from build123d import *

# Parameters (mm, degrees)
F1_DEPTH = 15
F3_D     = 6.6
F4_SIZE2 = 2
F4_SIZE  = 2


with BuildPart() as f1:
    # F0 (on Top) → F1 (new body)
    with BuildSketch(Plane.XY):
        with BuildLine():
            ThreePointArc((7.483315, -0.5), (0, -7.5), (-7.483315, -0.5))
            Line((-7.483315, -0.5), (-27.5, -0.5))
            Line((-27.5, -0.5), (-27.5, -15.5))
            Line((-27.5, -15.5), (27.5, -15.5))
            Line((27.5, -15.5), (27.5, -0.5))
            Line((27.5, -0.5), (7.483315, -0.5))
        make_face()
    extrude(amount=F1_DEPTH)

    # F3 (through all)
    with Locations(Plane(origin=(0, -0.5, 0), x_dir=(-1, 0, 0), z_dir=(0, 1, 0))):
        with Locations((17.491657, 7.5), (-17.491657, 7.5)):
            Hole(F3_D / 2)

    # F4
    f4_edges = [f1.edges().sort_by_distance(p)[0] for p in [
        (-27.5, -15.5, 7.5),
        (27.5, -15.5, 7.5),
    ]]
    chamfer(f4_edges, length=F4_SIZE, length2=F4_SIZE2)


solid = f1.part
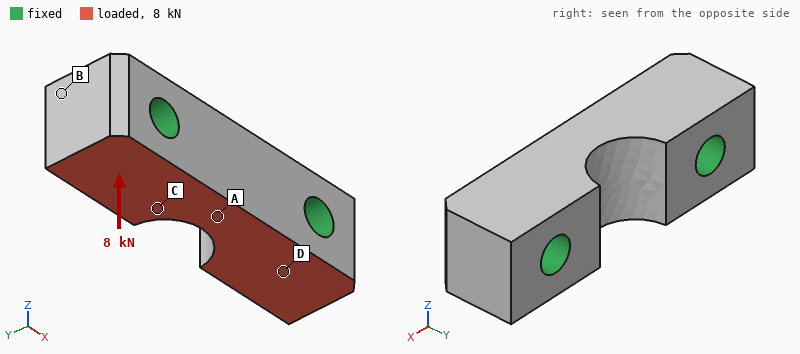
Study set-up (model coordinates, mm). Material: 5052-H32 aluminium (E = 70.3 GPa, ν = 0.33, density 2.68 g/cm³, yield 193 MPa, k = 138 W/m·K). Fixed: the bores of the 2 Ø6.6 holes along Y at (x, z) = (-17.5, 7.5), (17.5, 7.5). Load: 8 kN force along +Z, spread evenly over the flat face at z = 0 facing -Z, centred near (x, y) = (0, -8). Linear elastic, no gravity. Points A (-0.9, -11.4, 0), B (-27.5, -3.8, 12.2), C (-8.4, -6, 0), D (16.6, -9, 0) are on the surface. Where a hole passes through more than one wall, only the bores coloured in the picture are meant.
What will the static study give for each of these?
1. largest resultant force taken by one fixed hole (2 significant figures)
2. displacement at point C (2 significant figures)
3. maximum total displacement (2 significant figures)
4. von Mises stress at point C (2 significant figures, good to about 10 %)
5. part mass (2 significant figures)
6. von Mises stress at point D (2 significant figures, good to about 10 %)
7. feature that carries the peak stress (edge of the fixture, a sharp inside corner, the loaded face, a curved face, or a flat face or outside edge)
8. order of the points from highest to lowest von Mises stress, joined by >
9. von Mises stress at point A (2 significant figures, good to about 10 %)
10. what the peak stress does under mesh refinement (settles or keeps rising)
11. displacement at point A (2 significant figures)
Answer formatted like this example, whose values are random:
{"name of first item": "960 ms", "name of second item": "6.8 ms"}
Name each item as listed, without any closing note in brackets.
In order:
{"largest resultant force taken by one fixed hole": "4.0 kN", "displacement at point C": "4.2 µm", "maximum total displacement": "6.9 µm", "von Mises stress at point C": "9.1 MPa", "part mass": "27 g", "von Mises stress at point D": "25 MPa", "feature that carries the peak stress": "edge of the fixture", "order of the points from highest to lowest von Mises stress, joined by >": "D > A > C > B", "von Mises stress at point A": "16 MPa", "what the peak stress does under mesh refinement": "keeps rising", "displacement at point A": "6.0 µm"}
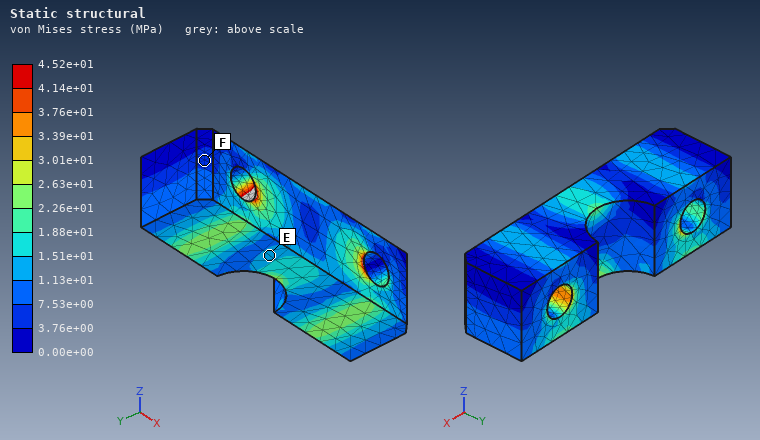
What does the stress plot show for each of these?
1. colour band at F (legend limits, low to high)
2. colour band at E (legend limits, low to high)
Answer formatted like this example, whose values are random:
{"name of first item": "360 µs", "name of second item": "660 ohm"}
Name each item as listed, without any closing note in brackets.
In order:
{"colour band at F": "3.76e+00 to 7.53e+00 MPa", "colour band at E": "1.13e+01 to 1.51e+01 MPa"}
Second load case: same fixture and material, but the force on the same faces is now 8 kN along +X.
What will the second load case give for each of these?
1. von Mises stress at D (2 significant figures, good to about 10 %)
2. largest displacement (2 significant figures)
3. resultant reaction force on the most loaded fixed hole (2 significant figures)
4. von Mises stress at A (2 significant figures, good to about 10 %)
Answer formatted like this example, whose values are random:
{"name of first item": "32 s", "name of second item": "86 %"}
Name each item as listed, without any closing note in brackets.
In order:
{"von Mises stress at D": "20 MPa", "largest displacement": "7.1 µm", "resultant reaction force on the most loaded fixed hole": "4.1 kN", "von Mises stress at A": "21 MPa"}
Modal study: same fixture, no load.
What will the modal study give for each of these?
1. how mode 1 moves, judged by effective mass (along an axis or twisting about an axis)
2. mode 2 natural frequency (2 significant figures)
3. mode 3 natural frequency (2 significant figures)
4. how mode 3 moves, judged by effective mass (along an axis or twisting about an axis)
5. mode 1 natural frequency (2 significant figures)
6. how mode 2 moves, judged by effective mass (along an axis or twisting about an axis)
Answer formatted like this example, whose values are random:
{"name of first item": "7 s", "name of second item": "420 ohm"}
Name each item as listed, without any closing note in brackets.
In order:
{"how mode 1 moves, judged by effective mass": "along Z", "mode 2 natural frequency": "44 kHz", "mode 3 natural frequency": "57 kHz", "how mode 3 moves, judged by effective mass": "twisting about X", "mode 1 natural frequency": "38 kHz", "how mode 2 moves, judged by effective mass": "along Y"}
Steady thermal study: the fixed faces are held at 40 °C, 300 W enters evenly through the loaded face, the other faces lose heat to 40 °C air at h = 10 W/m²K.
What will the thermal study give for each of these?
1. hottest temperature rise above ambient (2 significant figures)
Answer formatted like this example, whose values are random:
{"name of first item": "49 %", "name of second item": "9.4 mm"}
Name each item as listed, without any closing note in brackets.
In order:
{"hottest temperature rise above ambient": "37 K"}
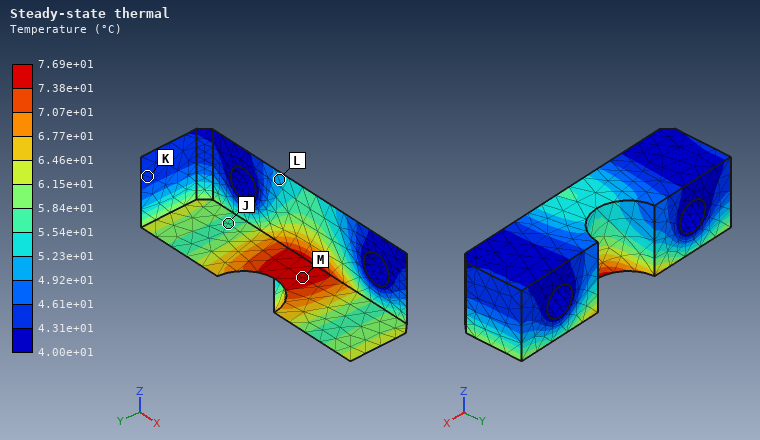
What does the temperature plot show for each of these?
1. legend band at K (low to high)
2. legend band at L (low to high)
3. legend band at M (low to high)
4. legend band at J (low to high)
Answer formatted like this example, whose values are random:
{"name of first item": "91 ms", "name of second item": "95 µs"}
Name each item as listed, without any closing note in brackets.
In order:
{"legend band at K": "4.31e+01 to 4.61e+01 °C", "legend band at L": "4.92e+01 to 5.23e+01 °C", "legend band at M": "7.38e+01 to 7.69e+01 °C", "legend band at J": "5.54e+01 to 5.84e+01 °C"}
